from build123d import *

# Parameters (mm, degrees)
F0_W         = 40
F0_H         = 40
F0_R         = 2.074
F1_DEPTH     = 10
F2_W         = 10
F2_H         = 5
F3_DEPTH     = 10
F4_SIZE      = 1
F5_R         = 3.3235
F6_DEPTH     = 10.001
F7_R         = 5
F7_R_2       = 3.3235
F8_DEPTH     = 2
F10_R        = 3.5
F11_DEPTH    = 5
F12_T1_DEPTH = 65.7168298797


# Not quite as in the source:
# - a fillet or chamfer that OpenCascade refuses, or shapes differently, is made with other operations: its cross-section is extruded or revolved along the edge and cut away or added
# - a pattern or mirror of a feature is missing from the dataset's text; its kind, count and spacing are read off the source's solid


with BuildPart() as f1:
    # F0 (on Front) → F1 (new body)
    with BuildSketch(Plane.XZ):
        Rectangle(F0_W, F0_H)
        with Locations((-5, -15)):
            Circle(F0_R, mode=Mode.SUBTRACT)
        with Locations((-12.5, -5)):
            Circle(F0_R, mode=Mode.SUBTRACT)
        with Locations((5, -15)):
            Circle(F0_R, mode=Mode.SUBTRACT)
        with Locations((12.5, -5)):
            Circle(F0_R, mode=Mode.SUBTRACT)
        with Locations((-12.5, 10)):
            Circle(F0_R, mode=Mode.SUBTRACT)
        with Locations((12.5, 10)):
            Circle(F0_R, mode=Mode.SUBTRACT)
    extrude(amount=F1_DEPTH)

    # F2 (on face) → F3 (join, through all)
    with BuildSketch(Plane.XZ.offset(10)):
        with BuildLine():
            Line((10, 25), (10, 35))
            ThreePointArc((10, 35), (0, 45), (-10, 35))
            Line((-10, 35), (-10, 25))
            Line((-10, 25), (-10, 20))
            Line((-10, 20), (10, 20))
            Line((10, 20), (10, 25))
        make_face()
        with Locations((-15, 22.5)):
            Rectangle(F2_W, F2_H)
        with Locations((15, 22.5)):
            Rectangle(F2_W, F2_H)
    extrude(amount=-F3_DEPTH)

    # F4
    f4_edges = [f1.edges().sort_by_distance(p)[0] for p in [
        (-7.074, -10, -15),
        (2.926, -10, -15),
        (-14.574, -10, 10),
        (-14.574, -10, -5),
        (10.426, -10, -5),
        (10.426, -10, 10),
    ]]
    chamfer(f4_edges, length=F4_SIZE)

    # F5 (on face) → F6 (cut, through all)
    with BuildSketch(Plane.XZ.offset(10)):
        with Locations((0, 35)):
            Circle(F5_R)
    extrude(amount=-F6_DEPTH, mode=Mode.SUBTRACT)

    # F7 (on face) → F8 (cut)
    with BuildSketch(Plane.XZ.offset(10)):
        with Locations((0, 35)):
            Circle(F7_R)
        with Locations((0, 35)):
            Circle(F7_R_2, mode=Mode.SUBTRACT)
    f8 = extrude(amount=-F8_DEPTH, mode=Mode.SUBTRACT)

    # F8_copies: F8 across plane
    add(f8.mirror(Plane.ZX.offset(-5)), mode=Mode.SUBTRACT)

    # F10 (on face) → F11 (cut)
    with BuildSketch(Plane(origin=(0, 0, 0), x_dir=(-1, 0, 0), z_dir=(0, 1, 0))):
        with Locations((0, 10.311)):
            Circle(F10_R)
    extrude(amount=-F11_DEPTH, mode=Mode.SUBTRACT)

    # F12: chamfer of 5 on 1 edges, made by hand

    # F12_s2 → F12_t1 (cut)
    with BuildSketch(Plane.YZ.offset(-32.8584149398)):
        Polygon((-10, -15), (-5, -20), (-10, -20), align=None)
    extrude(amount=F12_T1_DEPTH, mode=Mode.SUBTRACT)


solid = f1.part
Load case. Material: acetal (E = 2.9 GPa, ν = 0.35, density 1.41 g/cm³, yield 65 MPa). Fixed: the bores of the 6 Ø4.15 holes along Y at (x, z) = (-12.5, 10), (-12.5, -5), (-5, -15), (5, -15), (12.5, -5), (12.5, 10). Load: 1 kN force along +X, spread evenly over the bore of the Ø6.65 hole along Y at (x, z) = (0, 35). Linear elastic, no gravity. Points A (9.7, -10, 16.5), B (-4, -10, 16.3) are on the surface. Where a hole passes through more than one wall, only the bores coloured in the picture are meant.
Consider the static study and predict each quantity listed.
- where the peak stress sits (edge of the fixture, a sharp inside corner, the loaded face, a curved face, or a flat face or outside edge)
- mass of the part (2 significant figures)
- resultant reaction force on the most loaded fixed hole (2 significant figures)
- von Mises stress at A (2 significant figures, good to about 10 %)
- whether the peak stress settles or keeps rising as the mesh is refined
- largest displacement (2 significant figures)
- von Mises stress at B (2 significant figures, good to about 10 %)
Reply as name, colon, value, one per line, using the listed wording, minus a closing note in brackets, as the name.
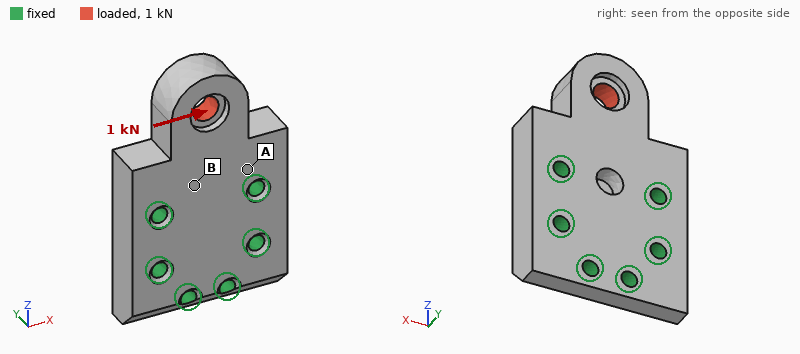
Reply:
where the peak stress sits: edge of the fixture
mass of the part: 28 g
resultant reaction force on the most loaded fixed hole: 930 N
von Mises stress at A: 9.6 MPa
whether the peak stress settles or keeps rising as the mesh is refined: keeps rising
largest displacement: 0.28 mm
von Mises stress at B: 4.1 MPa
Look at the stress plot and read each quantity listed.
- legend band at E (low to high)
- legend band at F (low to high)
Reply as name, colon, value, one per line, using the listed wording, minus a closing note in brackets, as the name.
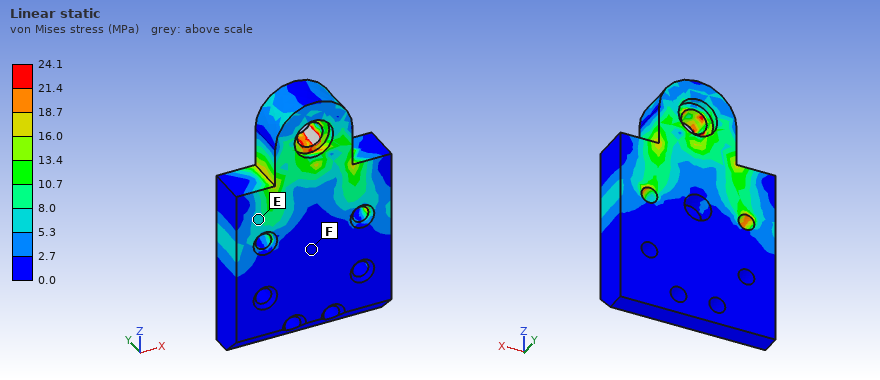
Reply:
legend band at E: 5.3 to 8.0 MPa
legend band at F: 0.0 to 2.7 MPa
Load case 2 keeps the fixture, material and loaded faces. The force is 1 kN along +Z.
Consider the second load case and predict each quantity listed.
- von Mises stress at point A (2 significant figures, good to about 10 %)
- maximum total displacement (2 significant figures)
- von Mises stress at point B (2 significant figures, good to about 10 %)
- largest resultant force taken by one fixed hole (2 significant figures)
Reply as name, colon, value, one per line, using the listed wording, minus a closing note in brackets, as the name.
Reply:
von Mises stress at point A: 4.2 MPa
maximum total displacement: 68 µm
von Mises stress at point B: 3.1 MPa
largest resultant force taken by one fixed hole: 410 N
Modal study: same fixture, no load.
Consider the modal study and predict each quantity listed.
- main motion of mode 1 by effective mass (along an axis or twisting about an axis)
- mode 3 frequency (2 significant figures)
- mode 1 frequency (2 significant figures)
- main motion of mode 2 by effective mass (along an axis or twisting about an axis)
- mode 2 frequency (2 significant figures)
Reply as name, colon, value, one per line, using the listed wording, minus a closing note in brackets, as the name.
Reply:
main motion of mode 1 by effective mass: along Y
mode 3 frequency: 6400 Hz
mode 1 frequency: 2300 Hz
main motion of mode 2 by effective mass: along X
mode 2 frequency: 5300 Hz
